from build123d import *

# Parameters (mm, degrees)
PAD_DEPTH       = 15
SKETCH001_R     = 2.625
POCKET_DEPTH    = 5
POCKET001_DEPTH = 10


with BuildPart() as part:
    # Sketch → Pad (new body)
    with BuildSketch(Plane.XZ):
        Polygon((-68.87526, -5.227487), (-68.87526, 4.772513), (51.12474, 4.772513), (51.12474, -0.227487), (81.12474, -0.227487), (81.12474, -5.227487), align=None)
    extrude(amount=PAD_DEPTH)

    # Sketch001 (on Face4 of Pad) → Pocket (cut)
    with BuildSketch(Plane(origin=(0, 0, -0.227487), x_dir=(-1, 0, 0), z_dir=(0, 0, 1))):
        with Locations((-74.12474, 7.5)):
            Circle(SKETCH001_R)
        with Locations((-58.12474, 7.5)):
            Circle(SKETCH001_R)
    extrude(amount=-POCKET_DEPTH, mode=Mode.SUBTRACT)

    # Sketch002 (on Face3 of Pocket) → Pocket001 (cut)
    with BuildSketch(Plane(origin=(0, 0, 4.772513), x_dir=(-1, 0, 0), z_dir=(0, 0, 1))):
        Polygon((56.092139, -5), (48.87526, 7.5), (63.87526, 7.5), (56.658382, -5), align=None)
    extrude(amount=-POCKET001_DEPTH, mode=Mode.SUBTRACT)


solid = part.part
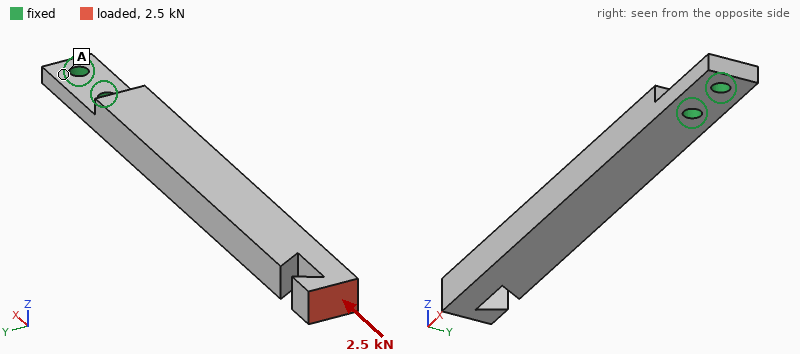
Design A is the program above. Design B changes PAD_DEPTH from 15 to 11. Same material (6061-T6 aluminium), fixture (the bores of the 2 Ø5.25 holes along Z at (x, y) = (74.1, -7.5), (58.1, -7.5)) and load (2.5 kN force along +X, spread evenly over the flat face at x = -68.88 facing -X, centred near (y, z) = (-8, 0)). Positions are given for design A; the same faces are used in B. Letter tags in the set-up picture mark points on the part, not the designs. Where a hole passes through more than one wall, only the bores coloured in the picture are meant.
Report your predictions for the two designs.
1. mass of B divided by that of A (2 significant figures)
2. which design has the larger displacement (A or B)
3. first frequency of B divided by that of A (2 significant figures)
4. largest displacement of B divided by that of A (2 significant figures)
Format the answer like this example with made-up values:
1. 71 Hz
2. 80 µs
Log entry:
1. 0.72
2. B
3. 1.0
4. 2.4
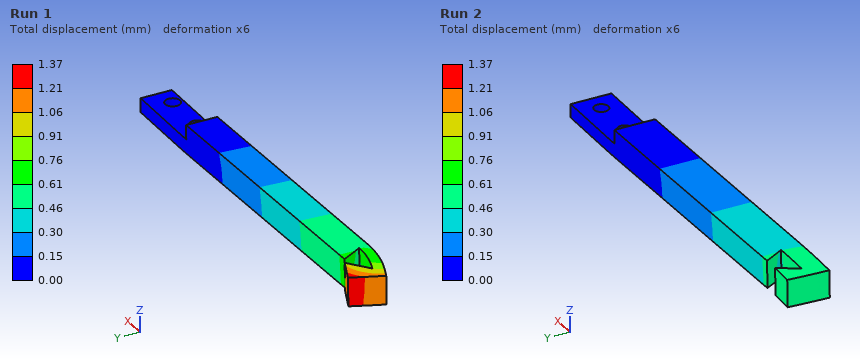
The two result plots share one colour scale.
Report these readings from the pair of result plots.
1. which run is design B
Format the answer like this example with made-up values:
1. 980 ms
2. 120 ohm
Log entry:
1. Run 1
